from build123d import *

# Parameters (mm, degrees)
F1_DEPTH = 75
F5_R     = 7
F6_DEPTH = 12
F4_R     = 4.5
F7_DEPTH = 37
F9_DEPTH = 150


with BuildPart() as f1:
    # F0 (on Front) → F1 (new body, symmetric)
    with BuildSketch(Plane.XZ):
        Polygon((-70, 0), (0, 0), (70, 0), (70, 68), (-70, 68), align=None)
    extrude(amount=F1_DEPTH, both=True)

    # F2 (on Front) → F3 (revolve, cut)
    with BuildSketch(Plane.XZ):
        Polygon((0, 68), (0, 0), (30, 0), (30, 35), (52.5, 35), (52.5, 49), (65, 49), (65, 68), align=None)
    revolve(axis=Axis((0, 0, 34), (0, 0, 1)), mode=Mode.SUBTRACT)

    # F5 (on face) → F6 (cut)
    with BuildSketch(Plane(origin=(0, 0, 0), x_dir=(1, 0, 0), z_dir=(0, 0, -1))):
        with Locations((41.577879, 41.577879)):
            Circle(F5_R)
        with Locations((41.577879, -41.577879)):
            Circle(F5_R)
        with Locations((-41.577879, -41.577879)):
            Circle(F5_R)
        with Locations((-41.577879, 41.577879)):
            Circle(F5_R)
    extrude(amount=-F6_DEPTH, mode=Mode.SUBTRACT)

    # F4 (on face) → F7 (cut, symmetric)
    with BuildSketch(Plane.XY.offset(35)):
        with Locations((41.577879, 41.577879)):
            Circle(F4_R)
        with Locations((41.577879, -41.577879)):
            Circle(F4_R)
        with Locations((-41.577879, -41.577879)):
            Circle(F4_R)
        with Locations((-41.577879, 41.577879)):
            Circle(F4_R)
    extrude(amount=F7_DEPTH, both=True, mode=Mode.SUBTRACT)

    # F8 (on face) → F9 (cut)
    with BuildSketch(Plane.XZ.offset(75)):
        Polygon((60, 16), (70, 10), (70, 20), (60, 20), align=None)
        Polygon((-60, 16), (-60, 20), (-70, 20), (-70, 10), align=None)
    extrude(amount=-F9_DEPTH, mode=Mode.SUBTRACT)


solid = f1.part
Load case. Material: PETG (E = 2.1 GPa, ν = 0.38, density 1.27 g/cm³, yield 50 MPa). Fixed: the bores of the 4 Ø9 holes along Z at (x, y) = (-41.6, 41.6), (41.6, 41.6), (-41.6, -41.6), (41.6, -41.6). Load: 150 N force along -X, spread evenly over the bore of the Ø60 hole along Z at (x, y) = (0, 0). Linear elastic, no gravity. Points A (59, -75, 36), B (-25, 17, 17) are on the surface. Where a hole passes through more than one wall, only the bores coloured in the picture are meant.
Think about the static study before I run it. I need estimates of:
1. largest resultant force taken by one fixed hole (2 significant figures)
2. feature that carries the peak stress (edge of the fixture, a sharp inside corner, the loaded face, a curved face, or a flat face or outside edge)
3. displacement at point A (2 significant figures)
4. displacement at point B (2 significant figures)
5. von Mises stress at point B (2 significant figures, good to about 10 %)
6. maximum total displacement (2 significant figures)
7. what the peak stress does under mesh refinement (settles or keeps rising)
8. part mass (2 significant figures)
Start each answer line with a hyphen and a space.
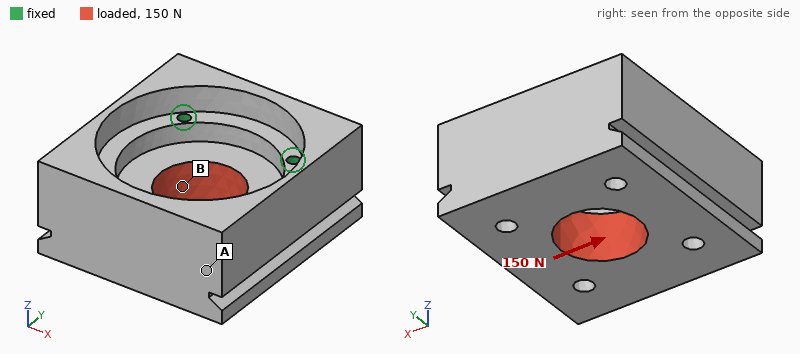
- 38 N
- edge of the fixture
- 0.20 µm
- 0.84 µm
- 0.025 MPa
- 1.3 µm
- keeps rising
- 1.2 kg
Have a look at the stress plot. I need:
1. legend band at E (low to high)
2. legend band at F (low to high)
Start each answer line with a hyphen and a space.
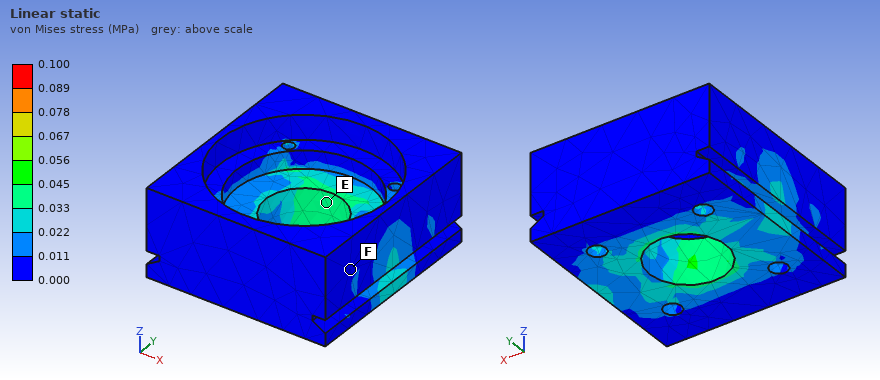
- 0.033 to 0.045 MPa
- 0.000 to 0.011 MPa
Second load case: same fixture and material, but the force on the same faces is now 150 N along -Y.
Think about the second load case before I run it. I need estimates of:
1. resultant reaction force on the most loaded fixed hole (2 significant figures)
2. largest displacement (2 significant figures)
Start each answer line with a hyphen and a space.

- 38 N
- 1.1 µm
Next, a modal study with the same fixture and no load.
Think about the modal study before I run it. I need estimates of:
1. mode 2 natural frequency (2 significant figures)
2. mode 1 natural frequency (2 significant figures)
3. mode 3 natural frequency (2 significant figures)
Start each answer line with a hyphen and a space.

- 2200 Hz
- 2200 Hz
- 2400 Hz
